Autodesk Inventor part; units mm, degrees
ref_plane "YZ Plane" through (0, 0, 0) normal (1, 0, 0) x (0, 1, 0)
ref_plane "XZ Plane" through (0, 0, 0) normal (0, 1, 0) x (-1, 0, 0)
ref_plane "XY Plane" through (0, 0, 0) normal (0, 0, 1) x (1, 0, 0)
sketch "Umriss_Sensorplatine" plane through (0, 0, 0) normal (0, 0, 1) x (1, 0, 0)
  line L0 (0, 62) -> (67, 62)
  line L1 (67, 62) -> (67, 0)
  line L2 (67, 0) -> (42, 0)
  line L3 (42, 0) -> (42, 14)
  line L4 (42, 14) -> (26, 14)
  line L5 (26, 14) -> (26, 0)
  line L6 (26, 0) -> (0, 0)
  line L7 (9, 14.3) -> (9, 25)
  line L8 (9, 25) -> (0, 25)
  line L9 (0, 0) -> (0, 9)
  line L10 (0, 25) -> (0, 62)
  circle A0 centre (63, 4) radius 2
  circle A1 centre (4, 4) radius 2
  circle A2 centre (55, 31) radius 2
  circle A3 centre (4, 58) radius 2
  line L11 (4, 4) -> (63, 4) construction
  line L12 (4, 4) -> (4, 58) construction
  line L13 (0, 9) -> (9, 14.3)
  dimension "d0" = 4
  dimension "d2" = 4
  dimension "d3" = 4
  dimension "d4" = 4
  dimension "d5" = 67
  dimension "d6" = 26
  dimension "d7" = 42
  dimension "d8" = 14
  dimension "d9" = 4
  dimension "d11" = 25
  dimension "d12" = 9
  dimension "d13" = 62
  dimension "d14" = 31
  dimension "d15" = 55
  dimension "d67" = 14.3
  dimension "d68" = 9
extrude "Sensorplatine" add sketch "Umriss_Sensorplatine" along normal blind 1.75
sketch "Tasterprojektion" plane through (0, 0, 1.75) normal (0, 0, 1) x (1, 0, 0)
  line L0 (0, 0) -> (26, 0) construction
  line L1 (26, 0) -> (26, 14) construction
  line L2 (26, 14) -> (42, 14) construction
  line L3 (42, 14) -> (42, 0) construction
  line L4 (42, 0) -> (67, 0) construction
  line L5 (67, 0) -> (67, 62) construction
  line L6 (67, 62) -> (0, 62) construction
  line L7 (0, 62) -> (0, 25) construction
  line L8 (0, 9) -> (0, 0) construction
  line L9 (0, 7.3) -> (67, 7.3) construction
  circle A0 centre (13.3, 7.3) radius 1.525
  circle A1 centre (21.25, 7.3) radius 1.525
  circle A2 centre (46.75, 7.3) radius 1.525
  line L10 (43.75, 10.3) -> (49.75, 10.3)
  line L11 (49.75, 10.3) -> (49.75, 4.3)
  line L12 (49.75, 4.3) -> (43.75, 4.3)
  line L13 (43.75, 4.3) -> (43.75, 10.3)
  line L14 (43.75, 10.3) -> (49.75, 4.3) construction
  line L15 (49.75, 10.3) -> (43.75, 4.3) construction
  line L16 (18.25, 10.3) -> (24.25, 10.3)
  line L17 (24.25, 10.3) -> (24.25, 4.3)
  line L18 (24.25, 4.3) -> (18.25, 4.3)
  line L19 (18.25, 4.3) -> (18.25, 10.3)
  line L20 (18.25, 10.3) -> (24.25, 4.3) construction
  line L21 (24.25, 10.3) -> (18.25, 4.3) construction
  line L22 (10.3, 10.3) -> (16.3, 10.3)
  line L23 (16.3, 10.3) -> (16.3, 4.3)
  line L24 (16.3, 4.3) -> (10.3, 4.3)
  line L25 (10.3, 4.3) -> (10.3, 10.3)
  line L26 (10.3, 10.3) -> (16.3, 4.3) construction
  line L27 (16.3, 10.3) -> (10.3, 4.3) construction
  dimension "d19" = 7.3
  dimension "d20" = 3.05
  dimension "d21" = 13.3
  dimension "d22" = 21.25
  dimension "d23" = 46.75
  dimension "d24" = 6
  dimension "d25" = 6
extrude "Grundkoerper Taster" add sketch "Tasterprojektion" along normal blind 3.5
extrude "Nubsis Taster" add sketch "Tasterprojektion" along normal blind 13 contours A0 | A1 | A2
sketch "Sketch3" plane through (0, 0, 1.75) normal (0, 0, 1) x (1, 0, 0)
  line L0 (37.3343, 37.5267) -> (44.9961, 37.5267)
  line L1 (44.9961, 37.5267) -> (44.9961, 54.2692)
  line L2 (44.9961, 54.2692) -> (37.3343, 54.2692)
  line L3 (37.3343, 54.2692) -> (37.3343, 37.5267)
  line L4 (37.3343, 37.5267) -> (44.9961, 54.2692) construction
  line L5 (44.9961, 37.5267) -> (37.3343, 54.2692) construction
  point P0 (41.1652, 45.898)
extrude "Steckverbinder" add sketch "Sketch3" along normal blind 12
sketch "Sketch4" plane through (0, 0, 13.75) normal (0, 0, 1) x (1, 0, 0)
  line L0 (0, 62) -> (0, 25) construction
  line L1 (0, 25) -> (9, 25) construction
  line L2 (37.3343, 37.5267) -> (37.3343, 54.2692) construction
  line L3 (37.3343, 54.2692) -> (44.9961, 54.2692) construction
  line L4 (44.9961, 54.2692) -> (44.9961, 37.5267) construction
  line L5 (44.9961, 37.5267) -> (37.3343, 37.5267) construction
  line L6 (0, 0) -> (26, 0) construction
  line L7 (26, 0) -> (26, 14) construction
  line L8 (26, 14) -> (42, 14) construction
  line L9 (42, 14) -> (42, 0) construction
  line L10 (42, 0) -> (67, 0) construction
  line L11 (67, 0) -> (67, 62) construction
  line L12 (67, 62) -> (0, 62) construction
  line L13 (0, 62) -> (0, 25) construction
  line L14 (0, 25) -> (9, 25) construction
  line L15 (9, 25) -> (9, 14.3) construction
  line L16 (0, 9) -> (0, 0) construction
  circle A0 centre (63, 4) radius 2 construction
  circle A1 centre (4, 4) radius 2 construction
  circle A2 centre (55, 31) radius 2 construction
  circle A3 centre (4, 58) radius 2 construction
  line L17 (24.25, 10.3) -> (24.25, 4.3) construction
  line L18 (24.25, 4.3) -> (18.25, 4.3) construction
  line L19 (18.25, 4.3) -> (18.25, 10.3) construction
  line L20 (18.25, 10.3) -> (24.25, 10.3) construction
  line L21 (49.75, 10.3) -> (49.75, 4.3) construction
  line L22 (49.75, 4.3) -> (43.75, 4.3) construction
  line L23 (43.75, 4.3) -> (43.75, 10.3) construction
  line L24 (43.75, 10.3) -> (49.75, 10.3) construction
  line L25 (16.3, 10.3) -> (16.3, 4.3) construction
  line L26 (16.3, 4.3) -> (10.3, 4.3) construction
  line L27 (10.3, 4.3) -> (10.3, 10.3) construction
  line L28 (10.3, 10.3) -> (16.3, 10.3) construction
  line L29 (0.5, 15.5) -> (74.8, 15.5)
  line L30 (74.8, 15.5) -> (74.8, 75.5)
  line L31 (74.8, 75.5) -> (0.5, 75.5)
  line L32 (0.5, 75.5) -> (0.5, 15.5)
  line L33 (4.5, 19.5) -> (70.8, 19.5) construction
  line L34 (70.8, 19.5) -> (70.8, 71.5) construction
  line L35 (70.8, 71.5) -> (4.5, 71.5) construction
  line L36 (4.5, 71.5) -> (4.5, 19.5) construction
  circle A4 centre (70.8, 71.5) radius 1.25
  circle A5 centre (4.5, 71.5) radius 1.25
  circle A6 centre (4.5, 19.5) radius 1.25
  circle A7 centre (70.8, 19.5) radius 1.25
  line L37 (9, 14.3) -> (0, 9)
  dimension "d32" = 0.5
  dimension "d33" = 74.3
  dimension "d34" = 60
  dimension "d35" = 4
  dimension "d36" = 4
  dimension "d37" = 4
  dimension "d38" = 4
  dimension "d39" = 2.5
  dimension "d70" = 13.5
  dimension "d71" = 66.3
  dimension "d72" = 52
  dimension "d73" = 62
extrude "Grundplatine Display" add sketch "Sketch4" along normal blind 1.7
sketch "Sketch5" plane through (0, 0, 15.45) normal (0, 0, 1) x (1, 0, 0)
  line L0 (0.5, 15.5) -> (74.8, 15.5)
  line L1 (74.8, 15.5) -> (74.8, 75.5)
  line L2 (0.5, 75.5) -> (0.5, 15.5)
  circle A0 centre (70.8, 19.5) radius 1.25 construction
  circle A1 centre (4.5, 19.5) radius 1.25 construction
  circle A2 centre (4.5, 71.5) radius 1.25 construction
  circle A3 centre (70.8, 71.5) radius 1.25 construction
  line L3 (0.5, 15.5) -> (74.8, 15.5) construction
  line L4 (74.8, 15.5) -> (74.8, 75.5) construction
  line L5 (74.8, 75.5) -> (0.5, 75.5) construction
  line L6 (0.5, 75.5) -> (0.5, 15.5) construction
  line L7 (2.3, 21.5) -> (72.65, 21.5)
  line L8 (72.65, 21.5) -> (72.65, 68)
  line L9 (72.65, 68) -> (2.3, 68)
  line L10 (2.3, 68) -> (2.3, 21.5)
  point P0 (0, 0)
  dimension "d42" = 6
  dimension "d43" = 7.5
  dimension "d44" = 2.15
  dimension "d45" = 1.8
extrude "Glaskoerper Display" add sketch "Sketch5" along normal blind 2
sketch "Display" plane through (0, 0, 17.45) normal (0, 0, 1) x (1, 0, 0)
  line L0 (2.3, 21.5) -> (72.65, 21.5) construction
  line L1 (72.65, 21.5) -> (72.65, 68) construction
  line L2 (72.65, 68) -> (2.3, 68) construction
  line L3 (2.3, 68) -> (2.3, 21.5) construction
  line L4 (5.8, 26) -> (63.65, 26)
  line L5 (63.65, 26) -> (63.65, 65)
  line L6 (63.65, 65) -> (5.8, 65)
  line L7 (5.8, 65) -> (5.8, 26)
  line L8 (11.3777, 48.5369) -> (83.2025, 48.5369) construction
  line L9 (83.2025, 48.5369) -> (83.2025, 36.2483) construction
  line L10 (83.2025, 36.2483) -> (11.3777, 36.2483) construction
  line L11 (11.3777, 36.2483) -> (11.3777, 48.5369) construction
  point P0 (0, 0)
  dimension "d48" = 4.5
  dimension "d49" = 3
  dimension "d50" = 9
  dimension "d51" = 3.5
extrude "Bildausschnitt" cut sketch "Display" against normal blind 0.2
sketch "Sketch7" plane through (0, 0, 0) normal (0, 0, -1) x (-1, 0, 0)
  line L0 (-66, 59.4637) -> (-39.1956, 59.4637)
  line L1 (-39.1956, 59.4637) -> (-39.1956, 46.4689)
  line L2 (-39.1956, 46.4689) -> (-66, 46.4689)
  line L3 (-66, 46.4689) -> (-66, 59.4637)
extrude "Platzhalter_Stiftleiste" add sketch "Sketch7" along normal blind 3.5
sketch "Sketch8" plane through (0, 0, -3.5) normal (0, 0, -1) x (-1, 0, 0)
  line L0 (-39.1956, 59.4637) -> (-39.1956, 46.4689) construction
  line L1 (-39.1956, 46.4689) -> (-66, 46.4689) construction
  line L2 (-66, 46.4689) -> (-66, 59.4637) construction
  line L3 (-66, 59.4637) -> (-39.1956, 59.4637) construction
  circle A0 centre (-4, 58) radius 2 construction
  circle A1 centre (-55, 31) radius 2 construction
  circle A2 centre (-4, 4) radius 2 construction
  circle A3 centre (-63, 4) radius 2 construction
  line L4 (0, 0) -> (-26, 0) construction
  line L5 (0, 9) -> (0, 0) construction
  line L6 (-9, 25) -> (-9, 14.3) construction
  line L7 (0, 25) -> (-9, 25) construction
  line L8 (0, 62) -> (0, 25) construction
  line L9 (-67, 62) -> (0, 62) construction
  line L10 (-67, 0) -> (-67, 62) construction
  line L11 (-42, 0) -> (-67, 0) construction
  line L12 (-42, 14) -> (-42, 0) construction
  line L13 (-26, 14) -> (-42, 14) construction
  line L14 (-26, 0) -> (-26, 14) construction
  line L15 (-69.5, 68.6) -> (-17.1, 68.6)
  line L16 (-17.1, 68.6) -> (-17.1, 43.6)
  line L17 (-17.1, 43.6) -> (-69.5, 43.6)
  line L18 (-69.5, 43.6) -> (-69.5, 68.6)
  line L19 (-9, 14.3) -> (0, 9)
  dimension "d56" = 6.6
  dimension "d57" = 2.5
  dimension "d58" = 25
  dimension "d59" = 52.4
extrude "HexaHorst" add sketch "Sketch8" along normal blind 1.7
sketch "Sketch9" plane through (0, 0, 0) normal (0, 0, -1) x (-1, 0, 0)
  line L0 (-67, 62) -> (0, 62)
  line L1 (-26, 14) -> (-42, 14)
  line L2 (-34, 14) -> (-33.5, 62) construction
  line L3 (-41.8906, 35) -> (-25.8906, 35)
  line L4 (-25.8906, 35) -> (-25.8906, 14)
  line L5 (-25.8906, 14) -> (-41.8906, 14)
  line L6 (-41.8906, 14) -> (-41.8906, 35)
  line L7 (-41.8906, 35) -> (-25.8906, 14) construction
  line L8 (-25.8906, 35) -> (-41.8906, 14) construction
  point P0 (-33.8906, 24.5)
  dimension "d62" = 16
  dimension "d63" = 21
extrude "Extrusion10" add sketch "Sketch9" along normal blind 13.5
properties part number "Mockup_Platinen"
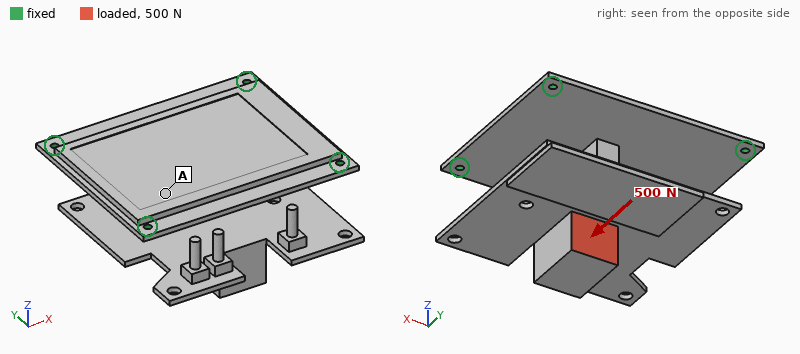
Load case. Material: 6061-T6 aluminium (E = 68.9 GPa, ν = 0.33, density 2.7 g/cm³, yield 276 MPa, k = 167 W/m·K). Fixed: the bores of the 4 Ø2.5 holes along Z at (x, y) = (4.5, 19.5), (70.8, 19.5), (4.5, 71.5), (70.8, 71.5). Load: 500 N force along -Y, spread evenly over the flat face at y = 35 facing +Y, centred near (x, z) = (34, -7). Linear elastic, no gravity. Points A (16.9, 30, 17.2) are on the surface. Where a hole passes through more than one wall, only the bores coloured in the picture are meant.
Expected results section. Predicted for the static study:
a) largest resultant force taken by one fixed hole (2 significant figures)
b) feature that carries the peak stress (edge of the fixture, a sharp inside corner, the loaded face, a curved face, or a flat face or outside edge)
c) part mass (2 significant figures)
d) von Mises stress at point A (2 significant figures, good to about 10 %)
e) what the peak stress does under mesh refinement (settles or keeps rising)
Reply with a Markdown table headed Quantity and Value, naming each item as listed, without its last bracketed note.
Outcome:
| Quantity | Value |
|---|---|
| largest resultant force taken by one fixed hole | 170 N |
| feature that carries the peak stress | edge of the fixture |
| part mass | 82 g |
| von Mises stress at point A | 22 MPa |
| what the peak stress does under mesh refinement | keeps rising |
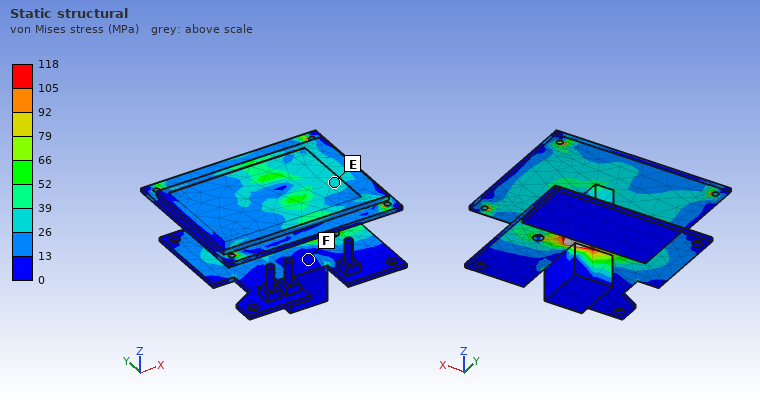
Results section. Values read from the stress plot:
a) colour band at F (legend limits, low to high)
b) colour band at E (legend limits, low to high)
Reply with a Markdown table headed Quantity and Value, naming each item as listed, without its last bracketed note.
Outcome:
| Quantity | Value |
|---|---|
| colour band at F | 0 to 13 MPa |
| colour band at E | 26 to 39 MPa |
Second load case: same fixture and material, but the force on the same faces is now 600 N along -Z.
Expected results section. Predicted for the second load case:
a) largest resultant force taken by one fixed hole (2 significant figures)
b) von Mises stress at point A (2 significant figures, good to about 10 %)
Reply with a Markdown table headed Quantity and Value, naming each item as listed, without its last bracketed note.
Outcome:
| Quantity | Value |
|---|---|
| largest resultant force taken by one fixed hole | 530 N |
| von Mises stress at point A | 29 MPa |
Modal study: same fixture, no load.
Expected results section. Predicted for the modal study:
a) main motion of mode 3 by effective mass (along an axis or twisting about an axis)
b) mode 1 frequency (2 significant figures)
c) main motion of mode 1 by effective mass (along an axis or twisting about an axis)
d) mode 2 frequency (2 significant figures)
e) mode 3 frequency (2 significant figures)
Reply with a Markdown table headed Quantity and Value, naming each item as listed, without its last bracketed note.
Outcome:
| Quantity | Value |
|---|---|
| main motion of mode 3 by effective mass | along Z |
| mode 1 frequency | 600 Hz |
| main motion of mode 1 by effective mass | along Z |
| mode 2 frequency | 960 Hz |
| mode 3 frequency | 1400 Hz |
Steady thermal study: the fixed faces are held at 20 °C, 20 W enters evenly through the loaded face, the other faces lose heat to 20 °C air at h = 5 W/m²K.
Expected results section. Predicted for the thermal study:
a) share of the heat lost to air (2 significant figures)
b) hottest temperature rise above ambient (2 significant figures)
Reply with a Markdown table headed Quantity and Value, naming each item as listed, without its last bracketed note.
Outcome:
| Quantity | Value |
|---|---|
| share of the heat lost to air | 14 % |
| hottest temperature rise above ambient | 55 K |
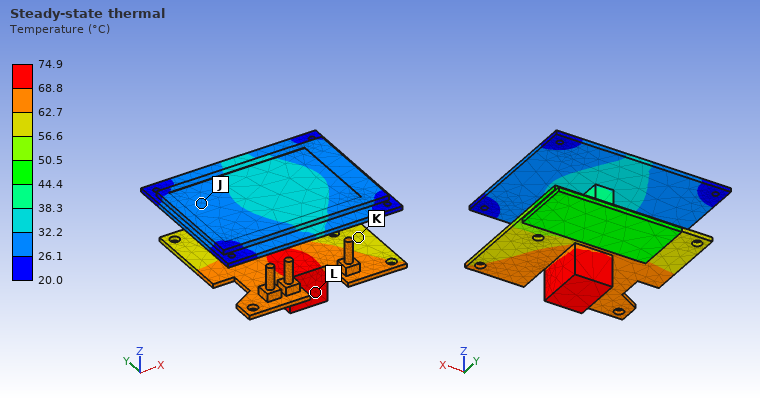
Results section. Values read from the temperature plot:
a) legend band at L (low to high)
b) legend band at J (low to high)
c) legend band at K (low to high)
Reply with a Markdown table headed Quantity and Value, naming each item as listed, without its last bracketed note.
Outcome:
| Quantity | Value |
|---|---|
| legend band at L | 68.8 to 74.9 °C |
| legend band at J | 26.1 to 32.2 °C |
| legend band at K | 56.6 to 62.7 °C |
